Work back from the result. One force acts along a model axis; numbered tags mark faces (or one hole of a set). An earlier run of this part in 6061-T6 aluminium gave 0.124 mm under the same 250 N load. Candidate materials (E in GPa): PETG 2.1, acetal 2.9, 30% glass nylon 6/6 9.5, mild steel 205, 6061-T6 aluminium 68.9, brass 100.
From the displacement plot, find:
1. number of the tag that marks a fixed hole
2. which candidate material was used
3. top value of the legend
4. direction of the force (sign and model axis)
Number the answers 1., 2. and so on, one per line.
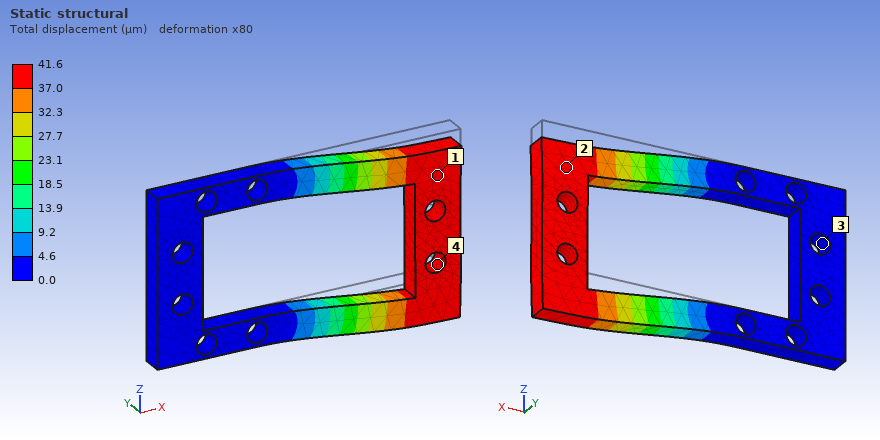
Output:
1. 3
2. mild steel
3. 41.6 µm
4. -Z
